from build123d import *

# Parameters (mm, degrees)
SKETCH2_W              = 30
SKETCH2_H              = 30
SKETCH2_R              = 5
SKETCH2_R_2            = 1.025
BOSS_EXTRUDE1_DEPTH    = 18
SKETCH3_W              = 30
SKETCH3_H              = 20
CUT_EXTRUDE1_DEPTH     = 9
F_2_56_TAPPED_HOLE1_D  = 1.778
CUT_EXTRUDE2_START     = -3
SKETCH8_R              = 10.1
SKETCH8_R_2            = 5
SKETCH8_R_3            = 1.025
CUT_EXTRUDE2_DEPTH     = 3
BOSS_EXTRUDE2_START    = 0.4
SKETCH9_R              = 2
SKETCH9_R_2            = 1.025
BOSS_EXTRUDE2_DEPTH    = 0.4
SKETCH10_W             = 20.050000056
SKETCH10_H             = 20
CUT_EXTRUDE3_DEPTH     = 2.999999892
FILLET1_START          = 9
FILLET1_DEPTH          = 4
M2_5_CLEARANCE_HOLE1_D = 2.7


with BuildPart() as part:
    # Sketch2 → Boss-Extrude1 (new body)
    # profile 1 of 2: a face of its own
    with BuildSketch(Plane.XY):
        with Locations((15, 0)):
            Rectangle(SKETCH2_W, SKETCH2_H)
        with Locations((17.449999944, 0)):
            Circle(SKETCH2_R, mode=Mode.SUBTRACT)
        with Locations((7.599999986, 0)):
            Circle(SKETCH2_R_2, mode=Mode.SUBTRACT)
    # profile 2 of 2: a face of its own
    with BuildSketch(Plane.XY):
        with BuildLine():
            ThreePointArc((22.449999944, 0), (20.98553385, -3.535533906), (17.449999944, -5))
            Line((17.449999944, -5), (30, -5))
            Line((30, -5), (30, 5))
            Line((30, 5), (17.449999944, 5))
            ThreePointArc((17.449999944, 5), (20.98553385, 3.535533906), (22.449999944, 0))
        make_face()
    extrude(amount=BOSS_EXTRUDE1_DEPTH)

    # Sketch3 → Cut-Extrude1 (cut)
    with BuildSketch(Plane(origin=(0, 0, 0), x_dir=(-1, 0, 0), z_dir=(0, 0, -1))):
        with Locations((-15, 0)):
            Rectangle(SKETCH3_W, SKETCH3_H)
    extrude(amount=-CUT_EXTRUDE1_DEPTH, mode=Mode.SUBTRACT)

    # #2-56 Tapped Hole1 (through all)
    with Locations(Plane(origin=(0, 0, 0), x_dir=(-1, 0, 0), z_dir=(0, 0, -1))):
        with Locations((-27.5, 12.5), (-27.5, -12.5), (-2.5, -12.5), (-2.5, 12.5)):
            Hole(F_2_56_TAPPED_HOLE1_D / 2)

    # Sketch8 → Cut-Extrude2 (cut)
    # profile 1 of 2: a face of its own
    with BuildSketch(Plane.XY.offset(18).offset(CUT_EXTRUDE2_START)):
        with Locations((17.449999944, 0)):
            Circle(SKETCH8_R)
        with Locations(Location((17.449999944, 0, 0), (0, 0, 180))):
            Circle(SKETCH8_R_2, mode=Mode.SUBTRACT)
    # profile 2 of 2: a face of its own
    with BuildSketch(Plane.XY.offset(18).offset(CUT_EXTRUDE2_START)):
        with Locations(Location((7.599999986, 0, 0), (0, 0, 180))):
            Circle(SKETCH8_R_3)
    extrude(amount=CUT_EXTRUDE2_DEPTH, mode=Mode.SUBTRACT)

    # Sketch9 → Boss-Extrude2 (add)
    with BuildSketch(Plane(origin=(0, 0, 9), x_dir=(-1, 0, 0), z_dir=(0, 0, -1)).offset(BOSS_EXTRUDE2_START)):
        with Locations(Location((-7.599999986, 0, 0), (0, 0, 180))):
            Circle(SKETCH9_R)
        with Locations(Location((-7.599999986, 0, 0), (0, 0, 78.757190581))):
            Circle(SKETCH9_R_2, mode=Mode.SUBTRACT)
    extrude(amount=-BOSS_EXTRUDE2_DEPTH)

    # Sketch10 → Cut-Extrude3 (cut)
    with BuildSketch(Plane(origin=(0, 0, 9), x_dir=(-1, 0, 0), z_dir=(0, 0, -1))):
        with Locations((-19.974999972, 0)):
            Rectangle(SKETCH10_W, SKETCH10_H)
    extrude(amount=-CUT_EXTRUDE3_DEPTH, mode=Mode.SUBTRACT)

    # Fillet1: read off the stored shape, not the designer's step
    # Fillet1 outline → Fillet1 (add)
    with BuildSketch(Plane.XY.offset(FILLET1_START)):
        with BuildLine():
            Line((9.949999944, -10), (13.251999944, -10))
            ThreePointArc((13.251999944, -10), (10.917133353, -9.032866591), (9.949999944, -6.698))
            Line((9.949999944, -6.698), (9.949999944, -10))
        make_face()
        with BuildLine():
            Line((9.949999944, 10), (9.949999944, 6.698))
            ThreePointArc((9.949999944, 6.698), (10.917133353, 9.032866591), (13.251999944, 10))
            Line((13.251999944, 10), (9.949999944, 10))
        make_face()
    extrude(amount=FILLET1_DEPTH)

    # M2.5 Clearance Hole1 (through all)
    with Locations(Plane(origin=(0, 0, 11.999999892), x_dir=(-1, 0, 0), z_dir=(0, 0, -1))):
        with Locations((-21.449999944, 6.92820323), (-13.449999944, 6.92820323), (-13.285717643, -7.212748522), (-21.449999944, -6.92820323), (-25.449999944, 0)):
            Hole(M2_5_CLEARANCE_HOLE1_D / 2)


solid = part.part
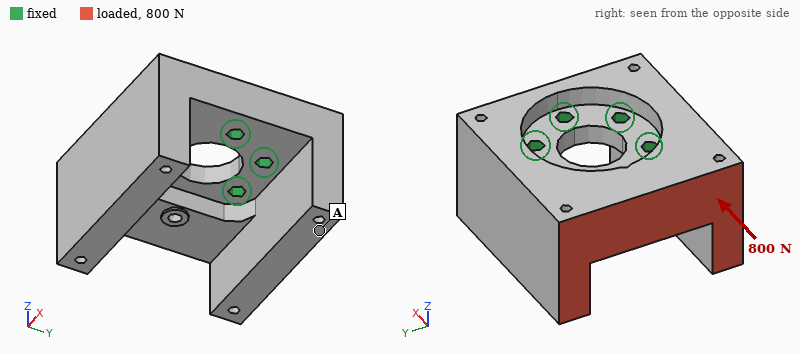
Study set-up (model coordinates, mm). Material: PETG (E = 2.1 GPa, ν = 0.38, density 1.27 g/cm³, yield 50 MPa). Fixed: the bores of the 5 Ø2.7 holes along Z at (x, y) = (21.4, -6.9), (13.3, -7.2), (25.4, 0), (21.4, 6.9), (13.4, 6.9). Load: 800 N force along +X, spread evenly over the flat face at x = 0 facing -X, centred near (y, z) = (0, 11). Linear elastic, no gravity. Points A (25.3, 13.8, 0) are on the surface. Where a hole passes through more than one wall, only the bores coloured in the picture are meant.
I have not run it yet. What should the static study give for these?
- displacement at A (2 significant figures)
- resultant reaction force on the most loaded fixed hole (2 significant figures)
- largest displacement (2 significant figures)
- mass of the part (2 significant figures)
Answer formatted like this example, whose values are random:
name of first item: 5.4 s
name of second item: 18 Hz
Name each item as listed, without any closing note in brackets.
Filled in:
displacement at A: 0.098 mm
resultant reaction force on the most loaded fixed hole: 310 N
largest displacement: 0.14 mm
mass of the part: 10 g
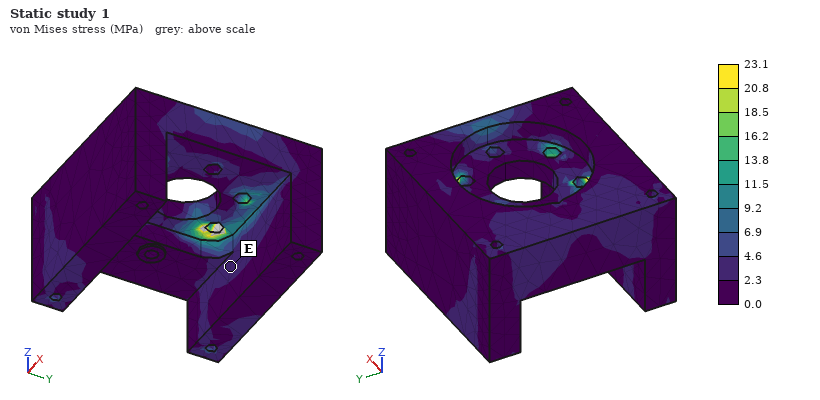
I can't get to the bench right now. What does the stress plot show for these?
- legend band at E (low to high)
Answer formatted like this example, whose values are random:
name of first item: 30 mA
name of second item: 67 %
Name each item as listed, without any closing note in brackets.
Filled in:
legend band at E: 2.3 to 4.6 MPa
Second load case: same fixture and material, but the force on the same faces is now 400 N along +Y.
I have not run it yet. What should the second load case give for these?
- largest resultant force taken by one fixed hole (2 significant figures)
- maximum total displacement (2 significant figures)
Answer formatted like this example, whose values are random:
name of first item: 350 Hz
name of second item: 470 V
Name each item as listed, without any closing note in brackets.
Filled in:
largest resultant force taken by one fixed hole: 310 N
maximum total displacement: 0.22 mm
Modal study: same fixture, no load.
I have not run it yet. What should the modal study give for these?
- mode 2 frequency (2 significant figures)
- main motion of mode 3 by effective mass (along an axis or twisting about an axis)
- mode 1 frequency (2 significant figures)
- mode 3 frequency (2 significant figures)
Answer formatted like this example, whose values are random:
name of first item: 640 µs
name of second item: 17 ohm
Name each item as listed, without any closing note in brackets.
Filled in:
mode 2 frequency: 2900 Hz
main motion of mode 3 by effective mass: along Z
mode 1 frequency: 2800 Hz
mode 3 frequency: 3400 Hz
